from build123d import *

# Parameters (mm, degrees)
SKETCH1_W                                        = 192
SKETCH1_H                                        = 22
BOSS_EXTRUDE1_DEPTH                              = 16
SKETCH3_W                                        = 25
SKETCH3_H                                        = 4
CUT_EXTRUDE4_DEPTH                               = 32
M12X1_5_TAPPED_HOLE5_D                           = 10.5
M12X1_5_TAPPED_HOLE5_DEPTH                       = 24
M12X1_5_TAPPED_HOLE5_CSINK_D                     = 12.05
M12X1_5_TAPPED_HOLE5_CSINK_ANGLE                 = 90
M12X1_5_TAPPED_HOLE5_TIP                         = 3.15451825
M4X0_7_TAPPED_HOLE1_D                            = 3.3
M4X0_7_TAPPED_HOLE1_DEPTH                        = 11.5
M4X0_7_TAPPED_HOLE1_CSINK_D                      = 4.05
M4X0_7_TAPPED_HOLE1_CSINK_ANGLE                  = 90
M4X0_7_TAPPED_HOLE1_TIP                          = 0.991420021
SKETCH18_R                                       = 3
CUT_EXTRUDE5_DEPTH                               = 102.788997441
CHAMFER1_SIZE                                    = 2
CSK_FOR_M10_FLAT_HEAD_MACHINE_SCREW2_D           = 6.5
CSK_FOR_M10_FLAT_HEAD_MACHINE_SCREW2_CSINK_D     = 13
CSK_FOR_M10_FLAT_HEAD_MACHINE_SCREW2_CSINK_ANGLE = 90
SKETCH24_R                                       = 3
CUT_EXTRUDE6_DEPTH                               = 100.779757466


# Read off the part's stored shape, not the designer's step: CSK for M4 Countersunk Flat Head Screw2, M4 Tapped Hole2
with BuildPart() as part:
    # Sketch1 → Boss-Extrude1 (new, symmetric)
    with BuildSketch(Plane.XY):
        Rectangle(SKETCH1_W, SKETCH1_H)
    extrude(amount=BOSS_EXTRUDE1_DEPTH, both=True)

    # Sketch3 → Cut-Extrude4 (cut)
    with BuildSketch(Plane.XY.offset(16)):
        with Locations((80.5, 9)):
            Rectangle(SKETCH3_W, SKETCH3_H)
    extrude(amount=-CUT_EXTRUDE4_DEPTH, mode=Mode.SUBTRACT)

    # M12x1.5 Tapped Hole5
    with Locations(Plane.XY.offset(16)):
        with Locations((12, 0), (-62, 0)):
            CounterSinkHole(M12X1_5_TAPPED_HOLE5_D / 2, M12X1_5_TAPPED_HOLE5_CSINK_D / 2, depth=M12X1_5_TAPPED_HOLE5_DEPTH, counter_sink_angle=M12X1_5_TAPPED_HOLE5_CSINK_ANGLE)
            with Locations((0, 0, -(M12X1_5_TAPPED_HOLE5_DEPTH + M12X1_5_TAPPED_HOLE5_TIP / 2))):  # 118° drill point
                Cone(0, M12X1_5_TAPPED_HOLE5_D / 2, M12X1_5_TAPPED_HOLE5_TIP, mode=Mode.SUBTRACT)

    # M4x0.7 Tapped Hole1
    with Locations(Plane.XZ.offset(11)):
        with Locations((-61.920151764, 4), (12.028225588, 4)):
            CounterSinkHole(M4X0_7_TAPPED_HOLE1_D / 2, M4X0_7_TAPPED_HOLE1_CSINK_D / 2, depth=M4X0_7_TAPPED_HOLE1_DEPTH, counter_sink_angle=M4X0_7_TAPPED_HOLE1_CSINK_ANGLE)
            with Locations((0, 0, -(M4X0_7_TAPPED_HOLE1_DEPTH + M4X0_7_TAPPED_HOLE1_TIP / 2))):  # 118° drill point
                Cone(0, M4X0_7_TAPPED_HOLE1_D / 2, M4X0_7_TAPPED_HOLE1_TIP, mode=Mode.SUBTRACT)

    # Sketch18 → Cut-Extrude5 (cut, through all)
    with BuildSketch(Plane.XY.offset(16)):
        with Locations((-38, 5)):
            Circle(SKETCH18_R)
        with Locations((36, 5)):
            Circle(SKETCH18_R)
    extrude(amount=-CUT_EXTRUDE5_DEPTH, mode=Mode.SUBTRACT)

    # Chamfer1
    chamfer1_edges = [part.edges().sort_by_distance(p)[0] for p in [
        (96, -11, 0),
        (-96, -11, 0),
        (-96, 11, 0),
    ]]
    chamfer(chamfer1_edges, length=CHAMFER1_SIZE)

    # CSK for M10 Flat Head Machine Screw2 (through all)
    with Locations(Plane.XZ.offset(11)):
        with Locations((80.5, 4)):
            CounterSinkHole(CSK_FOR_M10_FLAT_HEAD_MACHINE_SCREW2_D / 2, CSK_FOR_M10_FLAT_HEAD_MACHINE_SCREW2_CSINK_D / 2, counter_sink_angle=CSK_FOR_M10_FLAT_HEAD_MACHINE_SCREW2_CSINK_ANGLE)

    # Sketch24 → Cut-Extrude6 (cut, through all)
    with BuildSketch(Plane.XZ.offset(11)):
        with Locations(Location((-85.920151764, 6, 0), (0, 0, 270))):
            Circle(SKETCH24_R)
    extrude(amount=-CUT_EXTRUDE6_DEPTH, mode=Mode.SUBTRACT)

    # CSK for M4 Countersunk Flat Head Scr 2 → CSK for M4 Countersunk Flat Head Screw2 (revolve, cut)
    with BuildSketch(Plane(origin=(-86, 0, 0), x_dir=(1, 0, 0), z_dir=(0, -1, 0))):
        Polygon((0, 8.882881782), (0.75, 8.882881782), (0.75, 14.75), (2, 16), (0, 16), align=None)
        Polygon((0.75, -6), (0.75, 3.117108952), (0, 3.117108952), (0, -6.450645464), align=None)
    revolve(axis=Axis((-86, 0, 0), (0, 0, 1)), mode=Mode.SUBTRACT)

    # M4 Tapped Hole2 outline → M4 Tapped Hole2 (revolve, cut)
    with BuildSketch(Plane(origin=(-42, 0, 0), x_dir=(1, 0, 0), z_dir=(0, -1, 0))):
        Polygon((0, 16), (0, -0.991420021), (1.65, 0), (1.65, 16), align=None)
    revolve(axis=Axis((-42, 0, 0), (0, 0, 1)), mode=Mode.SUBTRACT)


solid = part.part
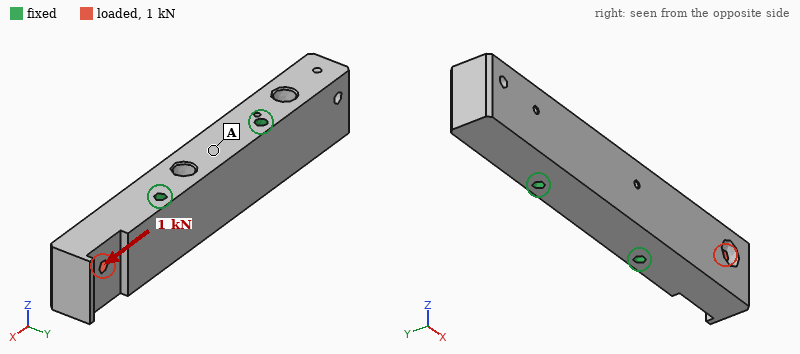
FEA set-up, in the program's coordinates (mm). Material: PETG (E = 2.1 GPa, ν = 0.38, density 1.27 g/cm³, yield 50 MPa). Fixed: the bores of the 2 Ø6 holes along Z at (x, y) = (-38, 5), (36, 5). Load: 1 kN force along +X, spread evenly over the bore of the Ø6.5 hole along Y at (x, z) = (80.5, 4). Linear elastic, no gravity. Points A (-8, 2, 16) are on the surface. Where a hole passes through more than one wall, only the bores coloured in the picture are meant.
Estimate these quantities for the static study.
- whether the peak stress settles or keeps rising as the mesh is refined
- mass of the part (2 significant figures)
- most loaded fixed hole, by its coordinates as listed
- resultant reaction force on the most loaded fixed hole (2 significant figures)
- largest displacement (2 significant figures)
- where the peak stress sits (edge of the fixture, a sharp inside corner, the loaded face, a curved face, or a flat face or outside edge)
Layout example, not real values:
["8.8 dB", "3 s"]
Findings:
["keeps rising", "160 g", "(36, 5)", "880 N", "0.10 mm", "edge of the fixture"]
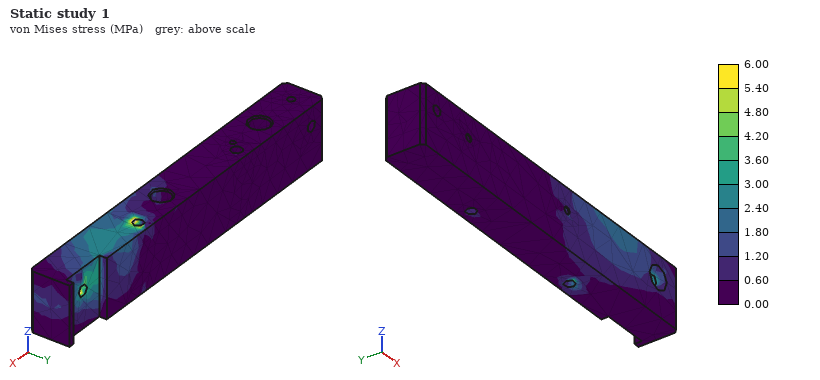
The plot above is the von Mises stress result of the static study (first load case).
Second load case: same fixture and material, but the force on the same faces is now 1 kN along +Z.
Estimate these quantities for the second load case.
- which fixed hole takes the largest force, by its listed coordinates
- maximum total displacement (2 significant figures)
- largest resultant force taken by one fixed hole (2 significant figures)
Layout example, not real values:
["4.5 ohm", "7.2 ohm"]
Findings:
["(36, 5)", "0.54 mm", "1.1 kN"]
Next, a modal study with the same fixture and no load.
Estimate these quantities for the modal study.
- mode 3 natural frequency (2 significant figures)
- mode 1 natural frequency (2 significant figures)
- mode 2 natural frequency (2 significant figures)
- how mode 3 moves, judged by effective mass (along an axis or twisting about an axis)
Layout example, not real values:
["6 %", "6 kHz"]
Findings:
["1500 Hz", "990 Hz", "1000 Hz", "along Z"]
